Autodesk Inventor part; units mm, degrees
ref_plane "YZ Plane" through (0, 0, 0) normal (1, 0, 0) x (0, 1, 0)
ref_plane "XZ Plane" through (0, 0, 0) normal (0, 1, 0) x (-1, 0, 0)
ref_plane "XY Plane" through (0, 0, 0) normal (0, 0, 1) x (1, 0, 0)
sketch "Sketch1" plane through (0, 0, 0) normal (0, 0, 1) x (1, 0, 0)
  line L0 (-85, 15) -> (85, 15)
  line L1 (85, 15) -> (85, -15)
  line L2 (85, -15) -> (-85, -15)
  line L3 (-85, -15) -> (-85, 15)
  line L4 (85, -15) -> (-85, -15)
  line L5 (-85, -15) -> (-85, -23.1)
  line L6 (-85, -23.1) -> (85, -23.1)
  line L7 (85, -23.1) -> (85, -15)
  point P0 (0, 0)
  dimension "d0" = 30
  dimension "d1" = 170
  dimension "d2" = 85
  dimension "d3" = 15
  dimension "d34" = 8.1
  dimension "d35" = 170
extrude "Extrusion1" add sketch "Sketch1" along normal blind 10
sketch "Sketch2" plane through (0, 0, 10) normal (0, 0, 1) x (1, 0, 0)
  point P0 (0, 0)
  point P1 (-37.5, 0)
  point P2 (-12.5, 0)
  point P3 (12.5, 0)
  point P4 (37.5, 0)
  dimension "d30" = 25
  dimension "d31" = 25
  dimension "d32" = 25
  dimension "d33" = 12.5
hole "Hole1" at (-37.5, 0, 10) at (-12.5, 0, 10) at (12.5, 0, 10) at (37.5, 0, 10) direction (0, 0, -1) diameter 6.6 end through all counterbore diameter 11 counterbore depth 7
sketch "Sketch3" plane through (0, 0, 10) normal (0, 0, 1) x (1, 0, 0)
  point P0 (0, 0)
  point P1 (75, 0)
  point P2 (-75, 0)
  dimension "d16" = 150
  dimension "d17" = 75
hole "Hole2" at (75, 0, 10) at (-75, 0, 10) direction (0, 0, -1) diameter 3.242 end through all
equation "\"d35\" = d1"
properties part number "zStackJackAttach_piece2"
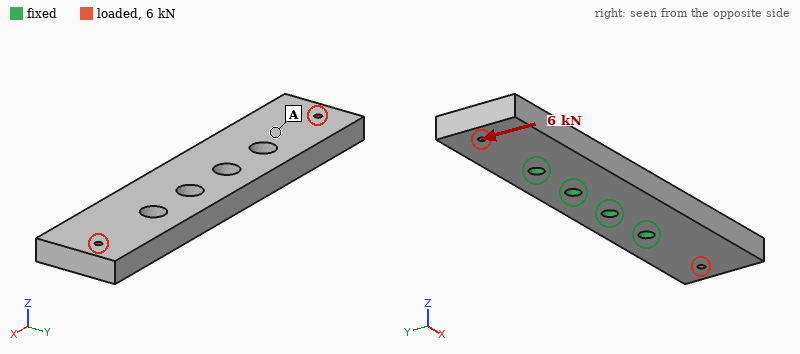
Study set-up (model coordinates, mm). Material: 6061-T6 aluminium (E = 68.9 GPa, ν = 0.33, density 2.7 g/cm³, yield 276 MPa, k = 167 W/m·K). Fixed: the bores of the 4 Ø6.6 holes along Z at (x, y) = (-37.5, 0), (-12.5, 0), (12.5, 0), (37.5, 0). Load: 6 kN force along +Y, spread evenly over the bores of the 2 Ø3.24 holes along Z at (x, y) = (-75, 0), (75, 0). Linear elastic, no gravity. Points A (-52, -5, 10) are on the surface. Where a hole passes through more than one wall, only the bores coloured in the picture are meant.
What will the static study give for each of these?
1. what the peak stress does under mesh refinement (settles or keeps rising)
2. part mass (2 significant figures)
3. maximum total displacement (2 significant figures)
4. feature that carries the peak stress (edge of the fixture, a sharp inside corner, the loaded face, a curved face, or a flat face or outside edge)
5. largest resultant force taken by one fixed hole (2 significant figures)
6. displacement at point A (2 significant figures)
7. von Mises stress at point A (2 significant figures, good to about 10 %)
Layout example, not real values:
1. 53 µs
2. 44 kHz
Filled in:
1. keeps rising
2. 170 g
3. 0.11 mm
4. edge of the fixture
5. 4.7 kN
6. 0.040 mm
7. 23 MPa
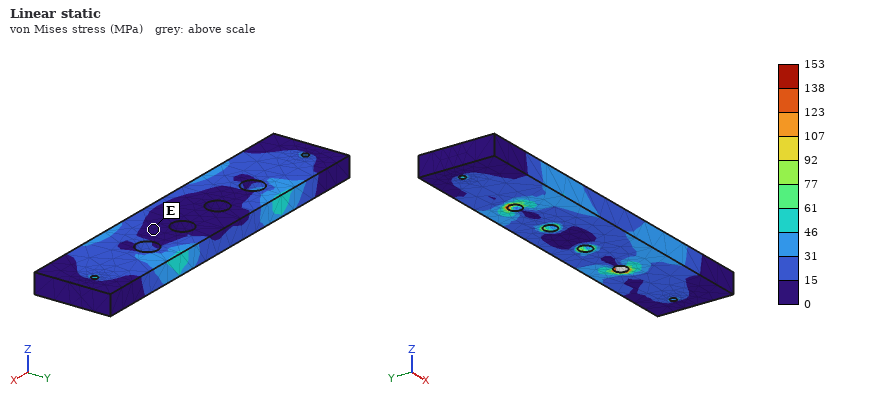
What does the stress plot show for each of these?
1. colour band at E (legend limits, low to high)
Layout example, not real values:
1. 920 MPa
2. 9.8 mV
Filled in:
1. 0 to 15 MPa
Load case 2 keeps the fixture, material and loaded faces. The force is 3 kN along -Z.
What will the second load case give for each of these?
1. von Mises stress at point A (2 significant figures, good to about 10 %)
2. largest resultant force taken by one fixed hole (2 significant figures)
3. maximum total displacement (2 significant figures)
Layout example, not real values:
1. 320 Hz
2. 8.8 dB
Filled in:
1. 46 MPa
2. 4.3 kN
3. 0.29 mm
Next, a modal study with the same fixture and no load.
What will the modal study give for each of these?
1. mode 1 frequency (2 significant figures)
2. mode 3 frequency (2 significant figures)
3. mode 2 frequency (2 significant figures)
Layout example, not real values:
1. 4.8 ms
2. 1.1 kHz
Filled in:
1. 2600 Hz
2. 4000 Hz
3. 2600 Hz
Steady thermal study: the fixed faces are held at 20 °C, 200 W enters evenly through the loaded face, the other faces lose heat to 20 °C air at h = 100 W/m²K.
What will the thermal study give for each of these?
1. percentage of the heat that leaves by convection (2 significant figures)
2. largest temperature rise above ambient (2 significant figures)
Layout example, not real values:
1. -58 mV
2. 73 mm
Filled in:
1. 25 %
2. 80 K
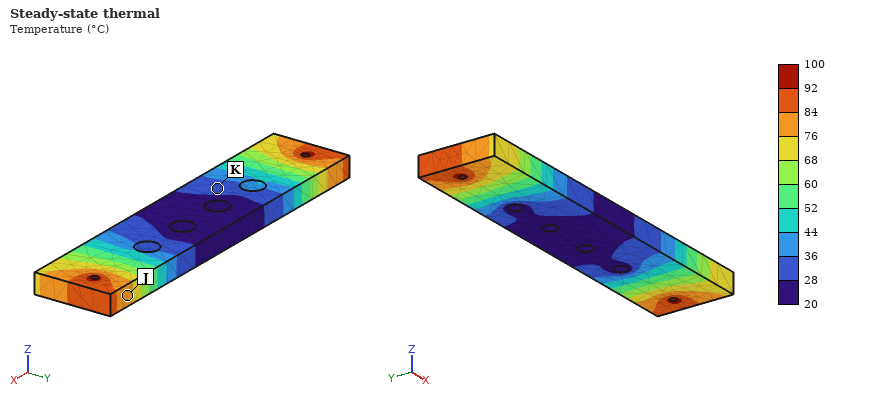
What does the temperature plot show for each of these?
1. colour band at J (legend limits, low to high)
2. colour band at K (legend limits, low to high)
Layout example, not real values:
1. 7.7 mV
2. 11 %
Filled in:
1. 76 to 84 °C
2. 28 to 36 °C
